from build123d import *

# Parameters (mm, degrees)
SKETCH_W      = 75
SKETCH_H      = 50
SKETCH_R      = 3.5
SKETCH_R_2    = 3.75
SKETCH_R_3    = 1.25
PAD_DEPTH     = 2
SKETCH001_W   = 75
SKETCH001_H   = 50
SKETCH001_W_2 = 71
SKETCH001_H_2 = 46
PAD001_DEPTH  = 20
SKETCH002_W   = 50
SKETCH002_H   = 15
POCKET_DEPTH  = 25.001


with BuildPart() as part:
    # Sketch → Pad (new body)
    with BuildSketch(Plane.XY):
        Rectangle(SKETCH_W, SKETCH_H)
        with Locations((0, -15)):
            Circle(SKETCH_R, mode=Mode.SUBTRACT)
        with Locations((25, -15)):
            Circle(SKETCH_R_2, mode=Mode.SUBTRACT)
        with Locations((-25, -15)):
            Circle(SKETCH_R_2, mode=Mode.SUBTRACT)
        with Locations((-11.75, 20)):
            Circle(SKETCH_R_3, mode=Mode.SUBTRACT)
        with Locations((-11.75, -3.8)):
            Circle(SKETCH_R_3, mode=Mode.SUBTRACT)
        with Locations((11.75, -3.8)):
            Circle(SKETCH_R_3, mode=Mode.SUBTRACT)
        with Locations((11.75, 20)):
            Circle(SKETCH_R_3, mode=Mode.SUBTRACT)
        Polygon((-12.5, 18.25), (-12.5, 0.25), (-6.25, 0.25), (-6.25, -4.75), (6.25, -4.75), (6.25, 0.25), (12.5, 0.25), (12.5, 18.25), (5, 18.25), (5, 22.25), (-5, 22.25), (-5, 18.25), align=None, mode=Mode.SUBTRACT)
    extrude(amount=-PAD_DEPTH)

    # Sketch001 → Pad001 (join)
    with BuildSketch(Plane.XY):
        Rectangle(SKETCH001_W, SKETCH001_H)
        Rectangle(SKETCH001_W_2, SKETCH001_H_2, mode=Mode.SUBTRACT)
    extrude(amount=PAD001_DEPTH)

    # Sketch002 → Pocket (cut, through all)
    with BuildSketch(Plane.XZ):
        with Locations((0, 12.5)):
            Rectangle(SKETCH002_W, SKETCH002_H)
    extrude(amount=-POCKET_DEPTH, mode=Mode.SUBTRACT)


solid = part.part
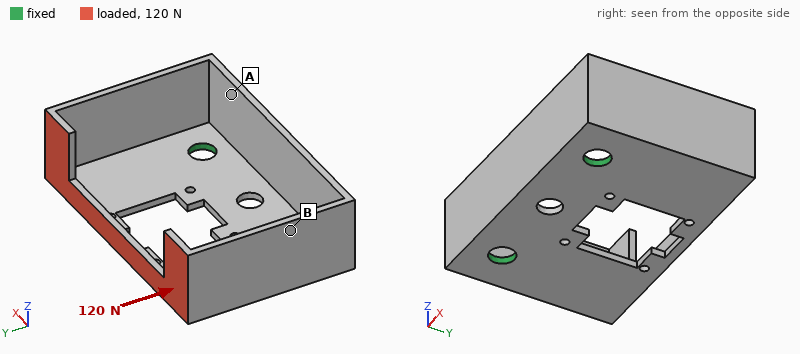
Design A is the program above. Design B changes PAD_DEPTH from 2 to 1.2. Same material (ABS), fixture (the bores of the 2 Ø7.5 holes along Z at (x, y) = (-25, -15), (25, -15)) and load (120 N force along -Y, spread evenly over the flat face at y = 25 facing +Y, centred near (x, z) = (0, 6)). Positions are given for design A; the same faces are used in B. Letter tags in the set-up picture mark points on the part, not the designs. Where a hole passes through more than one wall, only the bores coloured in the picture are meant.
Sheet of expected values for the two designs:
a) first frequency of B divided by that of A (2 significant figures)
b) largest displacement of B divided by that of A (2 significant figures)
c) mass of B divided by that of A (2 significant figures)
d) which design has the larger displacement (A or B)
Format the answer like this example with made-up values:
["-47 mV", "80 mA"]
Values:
["0.59", "2.9", "0.83", "B"]
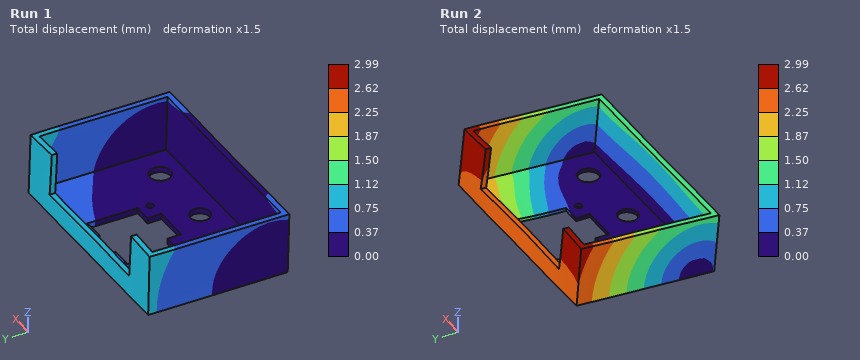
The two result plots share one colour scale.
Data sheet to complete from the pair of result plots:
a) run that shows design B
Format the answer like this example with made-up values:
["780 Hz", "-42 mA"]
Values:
["Run 2"]
